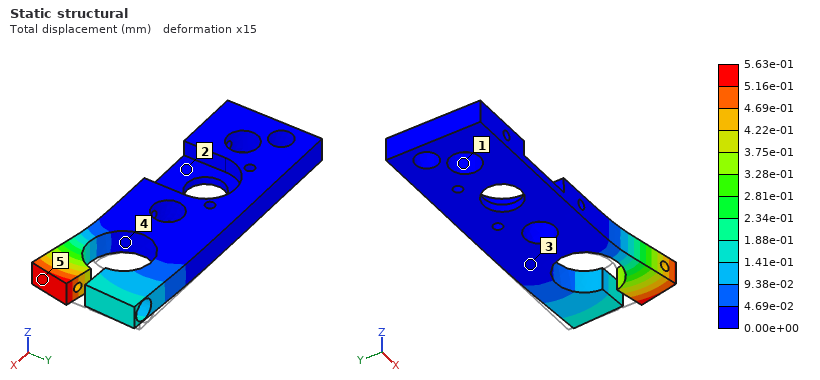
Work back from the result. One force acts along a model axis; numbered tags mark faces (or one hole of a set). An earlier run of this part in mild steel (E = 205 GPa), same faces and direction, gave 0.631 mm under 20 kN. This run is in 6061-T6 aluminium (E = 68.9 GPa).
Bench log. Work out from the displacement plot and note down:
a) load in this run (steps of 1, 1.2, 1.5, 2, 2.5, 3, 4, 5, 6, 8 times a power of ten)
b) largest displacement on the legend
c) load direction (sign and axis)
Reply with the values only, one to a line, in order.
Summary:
6 kN
5.63e-01 mm
-Y
